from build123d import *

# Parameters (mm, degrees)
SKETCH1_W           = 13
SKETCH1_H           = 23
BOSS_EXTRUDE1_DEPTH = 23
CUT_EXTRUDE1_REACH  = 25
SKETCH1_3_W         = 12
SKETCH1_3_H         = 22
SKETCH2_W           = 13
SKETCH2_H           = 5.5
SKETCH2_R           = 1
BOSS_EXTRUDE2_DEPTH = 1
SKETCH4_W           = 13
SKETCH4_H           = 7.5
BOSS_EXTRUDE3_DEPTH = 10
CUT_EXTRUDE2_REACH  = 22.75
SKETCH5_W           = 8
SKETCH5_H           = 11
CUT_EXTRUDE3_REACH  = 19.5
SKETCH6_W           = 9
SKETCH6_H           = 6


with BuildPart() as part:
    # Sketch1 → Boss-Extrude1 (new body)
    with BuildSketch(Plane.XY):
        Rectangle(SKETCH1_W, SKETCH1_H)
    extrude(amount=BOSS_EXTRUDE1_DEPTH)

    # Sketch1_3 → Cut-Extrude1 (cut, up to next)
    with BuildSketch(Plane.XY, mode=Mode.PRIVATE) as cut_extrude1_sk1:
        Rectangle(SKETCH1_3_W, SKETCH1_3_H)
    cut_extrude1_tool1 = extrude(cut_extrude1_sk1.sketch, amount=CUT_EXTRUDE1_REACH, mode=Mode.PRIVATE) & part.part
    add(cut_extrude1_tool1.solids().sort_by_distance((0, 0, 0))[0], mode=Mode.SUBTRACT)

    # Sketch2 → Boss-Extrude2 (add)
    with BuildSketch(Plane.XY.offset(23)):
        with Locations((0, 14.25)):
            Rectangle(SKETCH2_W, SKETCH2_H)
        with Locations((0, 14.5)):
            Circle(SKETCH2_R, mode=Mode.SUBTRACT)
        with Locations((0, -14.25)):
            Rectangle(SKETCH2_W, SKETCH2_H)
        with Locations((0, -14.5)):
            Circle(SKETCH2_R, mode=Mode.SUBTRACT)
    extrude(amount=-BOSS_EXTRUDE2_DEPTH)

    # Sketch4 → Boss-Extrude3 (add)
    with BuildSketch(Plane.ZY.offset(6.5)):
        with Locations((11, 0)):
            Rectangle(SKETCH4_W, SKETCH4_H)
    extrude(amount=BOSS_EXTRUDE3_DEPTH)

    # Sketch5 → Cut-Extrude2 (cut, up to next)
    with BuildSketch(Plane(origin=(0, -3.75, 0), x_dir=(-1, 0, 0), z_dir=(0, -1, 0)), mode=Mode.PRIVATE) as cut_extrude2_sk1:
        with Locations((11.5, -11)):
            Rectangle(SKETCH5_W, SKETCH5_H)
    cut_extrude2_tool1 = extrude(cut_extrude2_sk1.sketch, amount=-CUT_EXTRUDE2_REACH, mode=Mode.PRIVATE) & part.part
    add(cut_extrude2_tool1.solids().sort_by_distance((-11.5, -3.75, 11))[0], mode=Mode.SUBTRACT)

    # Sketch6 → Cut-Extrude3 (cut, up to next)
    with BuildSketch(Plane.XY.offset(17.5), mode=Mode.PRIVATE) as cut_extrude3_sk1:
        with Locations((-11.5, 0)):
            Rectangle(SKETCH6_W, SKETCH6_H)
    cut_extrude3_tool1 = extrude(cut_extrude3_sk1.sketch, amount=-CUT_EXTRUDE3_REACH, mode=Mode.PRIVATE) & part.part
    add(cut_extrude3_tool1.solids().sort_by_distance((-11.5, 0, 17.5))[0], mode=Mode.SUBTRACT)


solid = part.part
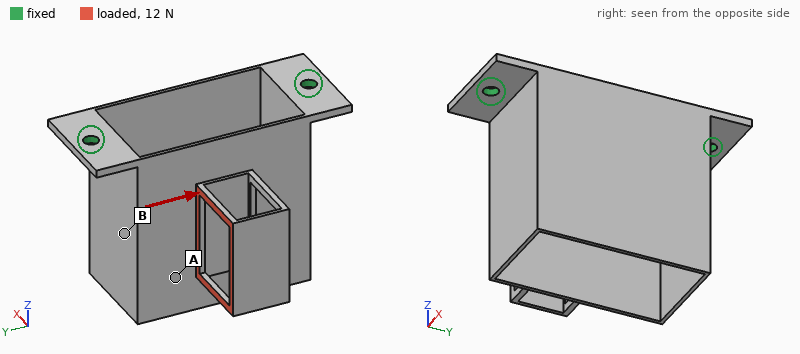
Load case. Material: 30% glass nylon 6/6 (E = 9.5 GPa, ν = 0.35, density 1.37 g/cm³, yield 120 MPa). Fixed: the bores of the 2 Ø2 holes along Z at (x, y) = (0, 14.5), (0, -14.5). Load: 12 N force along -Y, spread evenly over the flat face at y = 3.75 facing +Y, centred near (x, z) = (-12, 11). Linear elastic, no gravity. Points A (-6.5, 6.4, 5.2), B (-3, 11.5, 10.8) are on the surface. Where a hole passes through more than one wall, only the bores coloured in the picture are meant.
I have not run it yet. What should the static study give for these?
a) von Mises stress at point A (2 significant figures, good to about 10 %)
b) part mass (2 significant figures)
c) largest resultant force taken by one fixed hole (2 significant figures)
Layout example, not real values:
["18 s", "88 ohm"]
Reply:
["9.6 MPa", "1.5 g", "9.0 N"]
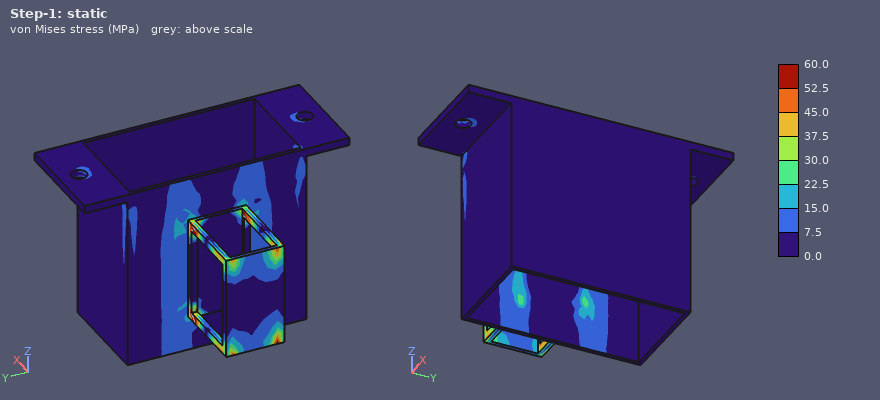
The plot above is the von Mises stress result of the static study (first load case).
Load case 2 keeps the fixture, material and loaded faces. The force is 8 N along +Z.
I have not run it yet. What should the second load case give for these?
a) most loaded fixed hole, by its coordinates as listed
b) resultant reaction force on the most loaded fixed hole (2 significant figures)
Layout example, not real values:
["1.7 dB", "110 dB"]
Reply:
["(0, 14.5)", "5.7 N"]
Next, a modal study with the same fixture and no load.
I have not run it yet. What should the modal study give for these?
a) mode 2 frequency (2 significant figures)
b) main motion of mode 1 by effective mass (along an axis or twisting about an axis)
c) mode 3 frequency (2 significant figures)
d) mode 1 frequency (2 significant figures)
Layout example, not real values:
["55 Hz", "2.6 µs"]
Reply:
["1600 Hz", "along X", "1800 Hz", "920 Hz"]
